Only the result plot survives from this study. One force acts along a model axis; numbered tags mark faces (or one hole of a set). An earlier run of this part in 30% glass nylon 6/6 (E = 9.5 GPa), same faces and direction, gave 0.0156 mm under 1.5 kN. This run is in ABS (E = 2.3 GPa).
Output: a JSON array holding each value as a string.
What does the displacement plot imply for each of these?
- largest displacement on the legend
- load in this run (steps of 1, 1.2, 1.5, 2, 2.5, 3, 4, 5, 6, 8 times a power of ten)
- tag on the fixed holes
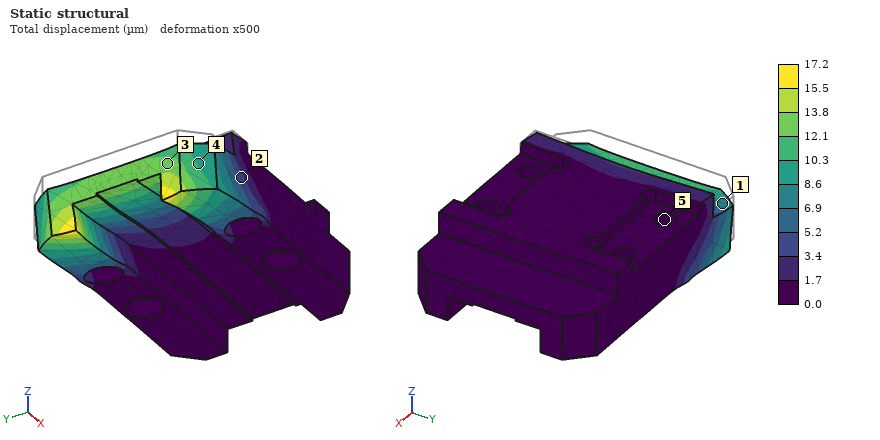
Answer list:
["17.2 µm", "400 N", "5"]
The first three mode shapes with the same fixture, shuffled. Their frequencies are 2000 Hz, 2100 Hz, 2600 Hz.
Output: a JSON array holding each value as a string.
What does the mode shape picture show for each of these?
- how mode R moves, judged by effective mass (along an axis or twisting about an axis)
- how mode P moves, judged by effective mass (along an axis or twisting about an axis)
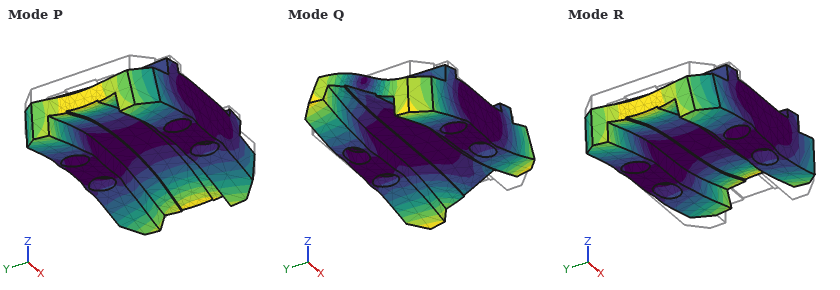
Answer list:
["twisting about Y", "along Z"]
